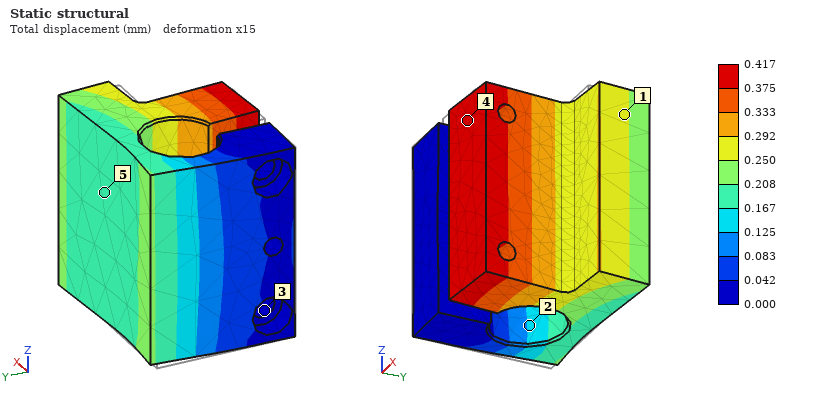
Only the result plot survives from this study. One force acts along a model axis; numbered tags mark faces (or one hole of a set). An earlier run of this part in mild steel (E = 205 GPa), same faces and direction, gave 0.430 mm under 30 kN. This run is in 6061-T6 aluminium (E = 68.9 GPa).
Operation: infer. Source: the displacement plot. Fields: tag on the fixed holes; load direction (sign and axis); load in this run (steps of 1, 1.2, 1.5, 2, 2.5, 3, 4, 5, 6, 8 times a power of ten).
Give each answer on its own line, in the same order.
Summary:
3
+X
10 kN
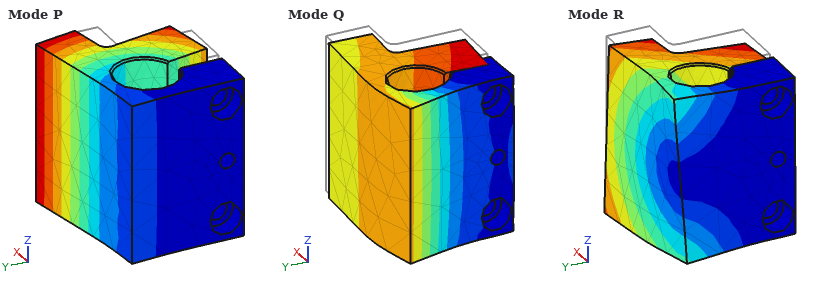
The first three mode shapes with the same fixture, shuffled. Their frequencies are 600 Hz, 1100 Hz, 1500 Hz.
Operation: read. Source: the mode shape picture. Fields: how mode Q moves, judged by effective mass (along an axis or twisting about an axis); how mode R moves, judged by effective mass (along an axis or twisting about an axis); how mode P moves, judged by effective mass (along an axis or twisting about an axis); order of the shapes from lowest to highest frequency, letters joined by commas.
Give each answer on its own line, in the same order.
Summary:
along X
along Z
along Y
P, R, Q
